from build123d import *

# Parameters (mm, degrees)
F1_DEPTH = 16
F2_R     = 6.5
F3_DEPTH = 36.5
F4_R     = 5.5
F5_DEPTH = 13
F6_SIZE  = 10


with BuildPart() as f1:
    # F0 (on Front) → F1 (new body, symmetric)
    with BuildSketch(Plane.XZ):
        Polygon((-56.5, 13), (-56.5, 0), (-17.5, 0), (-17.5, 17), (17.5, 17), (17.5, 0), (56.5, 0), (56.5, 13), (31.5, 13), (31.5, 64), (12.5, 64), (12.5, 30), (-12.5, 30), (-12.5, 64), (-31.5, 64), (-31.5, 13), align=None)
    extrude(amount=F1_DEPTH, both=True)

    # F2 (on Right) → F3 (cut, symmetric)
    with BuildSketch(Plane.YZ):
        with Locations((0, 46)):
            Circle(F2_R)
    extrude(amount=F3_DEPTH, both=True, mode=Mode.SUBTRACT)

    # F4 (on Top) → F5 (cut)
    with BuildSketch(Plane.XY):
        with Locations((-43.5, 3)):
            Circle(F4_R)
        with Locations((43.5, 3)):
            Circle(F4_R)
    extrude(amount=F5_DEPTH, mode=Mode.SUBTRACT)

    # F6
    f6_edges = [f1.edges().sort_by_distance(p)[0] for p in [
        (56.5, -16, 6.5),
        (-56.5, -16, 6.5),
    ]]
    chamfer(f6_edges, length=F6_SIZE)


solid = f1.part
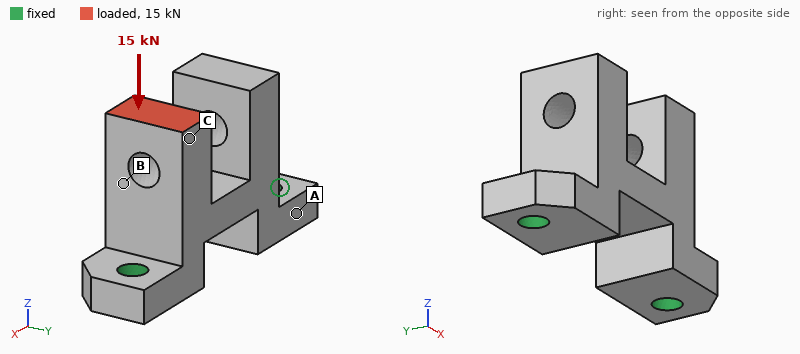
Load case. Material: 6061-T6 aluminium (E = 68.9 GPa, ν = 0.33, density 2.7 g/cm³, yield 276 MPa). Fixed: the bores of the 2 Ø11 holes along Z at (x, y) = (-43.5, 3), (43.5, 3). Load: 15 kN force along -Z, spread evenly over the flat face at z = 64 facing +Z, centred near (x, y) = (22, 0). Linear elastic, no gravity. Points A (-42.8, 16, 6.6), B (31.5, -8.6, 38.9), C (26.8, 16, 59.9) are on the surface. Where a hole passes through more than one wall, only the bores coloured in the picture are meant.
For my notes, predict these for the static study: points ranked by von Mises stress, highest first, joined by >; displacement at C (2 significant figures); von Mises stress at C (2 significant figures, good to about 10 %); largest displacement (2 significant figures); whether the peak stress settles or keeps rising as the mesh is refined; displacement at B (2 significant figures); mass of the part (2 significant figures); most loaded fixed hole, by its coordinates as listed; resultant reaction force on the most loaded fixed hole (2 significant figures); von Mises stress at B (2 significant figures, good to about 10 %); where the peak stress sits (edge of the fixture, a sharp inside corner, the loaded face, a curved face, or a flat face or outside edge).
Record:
B > C > A
56 µm
26 MPa
74 µm
keeps rising
58 µm
260 g
(43.5, 3)
13 kN
44 MPa
edge of the fixture
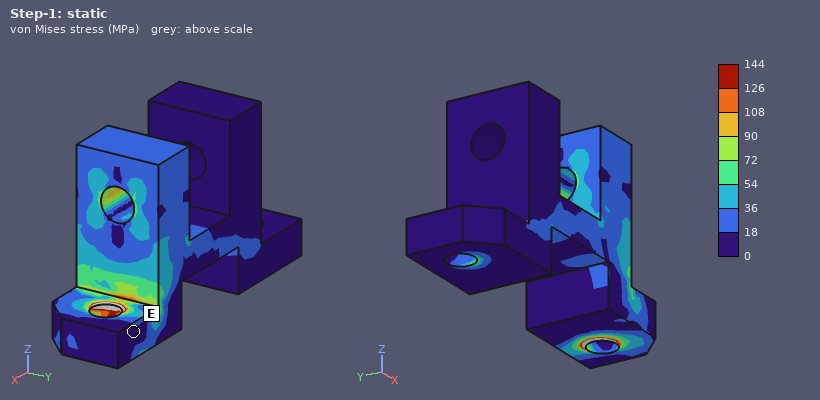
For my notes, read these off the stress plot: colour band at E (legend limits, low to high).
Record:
0 to 18 MPa
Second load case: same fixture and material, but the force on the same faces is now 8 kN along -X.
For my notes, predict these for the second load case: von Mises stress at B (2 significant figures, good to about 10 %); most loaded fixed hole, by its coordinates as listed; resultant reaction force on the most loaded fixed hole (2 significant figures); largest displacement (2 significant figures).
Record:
160 MPa
(-43.5, 3)
12 kN
0.35 mm
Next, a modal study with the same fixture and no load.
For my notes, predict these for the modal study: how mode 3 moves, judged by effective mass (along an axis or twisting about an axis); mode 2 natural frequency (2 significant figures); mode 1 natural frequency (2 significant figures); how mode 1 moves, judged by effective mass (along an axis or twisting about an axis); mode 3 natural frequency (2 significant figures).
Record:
along X
4500 Hz
2700 Hz
along Y
5400 Hz
